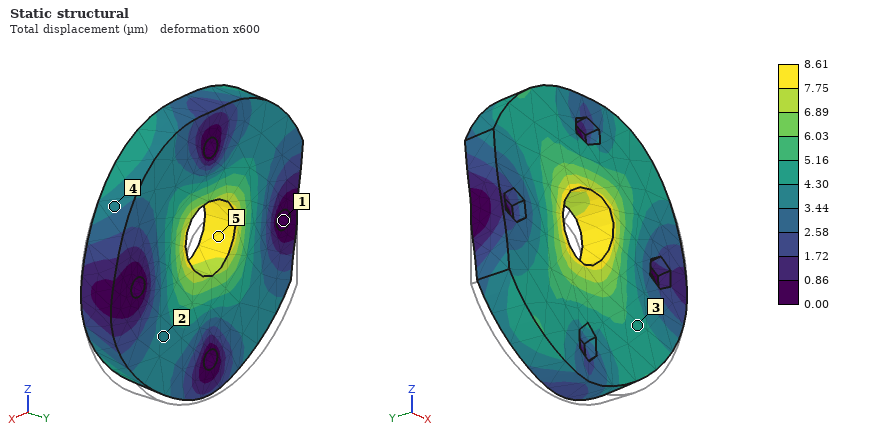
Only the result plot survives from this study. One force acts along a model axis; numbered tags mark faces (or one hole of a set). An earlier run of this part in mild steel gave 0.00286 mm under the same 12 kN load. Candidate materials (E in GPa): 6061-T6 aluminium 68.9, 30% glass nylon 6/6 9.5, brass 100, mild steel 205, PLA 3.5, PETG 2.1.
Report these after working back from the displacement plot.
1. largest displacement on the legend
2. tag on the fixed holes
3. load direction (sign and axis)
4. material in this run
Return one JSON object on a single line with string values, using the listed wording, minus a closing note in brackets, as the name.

{"largest displacement on the legend": "8.61 µm", "tag on the fixed holes": "1", "load direction": "+Z", "material in this run": "6061-T6 aluminium"}
